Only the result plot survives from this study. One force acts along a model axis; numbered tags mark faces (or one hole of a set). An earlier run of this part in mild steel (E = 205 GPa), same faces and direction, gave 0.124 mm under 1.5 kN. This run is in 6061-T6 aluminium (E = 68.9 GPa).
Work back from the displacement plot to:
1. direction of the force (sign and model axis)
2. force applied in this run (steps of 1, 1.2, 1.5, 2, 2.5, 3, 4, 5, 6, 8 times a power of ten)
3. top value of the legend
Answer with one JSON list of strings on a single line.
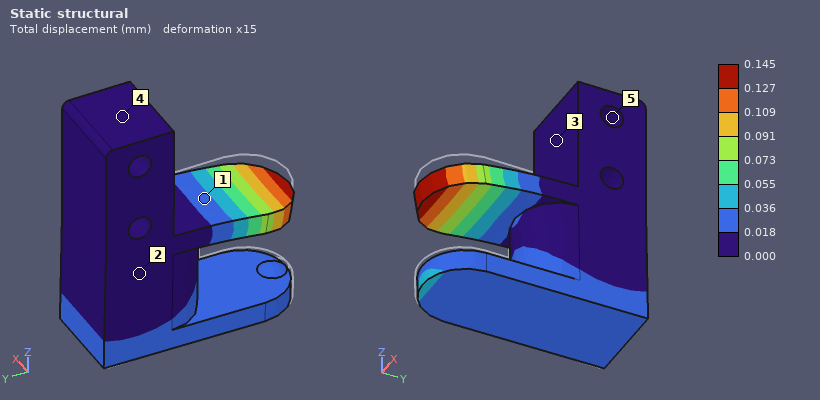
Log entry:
["-Z", "600 N", "0.145 mm"]
